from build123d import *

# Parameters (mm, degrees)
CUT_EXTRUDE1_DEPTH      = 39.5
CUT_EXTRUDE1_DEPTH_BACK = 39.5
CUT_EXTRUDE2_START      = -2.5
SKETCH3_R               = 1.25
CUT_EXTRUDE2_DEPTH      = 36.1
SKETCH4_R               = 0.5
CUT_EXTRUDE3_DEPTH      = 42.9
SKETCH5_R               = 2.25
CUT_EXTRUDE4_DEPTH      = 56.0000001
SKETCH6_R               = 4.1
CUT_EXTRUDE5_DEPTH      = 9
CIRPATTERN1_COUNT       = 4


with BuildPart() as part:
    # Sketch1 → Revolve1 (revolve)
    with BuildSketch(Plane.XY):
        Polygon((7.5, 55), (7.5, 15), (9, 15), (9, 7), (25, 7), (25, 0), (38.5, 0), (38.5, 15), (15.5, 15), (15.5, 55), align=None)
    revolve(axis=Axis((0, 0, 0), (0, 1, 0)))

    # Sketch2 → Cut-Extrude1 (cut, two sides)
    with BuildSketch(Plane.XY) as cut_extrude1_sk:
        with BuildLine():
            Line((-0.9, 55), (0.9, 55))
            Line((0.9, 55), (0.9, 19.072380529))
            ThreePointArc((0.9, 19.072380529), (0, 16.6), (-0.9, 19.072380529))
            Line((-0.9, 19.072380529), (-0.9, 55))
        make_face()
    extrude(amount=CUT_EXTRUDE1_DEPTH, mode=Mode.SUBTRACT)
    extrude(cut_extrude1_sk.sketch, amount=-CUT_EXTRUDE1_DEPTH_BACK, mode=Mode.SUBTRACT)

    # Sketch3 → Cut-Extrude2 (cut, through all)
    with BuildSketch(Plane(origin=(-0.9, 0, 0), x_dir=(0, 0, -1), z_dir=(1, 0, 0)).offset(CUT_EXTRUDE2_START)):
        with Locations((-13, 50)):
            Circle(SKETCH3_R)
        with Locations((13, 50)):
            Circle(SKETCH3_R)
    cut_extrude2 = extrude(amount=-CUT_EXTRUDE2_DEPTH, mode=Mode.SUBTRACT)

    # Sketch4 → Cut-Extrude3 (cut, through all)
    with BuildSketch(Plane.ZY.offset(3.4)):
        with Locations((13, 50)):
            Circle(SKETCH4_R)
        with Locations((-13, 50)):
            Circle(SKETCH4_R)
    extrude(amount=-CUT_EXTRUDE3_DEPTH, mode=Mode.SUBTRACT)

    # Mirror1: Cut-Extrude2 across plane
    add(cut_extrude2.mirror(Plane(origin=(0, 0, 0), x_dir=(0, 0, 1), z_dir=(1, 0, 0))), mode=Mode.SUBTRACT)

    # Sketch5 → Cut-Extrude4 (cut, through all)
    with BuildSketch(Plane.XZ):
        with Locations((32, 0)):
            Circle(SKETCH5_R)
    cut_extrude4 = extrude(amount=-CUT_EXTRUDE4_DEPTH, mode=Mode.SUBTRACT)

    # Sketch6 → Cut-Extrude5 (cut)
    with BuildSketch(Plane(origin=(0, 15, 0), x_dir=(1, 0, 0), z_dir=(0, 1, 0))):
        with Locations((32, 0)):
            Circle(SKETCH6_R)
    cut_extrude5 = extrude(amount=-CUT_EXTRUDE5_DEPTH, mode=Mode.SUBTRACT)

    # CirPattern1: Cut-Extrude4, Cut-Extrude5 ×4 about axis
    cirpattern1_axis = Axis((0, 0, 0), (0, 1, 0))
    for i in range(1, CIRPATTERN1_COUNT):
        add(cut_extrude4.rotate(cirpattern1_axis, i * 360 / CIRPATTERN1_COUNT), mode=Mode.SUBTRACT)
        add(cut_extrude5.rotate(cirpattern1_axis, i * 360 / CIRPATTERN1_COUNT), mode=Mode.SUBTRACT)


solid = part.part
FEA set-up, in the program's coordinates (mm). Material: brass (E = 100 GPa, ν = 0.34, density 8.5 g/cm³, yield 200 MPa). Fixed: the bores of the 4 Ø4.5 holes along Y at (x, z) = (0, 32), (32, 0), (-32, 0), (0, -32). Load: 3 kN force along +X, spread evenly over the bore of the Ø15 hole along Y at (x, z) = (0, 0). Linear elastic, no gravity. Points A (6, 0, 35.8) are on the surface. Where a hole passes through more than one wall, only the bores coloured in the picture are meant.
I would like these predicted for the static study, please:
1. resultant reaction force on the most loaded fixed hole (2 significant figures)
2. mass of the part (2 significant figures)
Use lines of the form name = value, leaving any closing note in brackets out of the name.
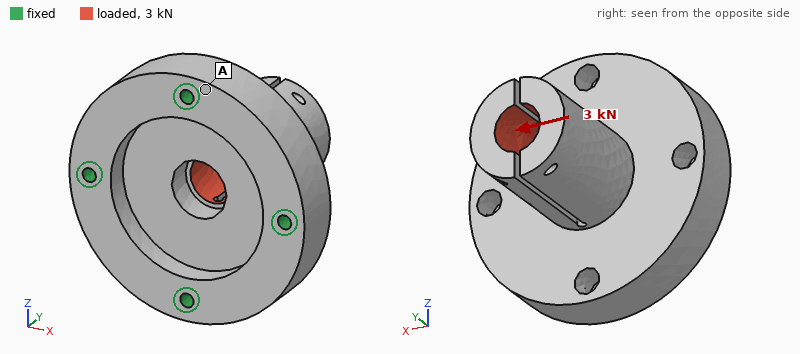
resultant reaction force on the most loaded fixed hole = 1.9 kN
mass of the part = 630 g
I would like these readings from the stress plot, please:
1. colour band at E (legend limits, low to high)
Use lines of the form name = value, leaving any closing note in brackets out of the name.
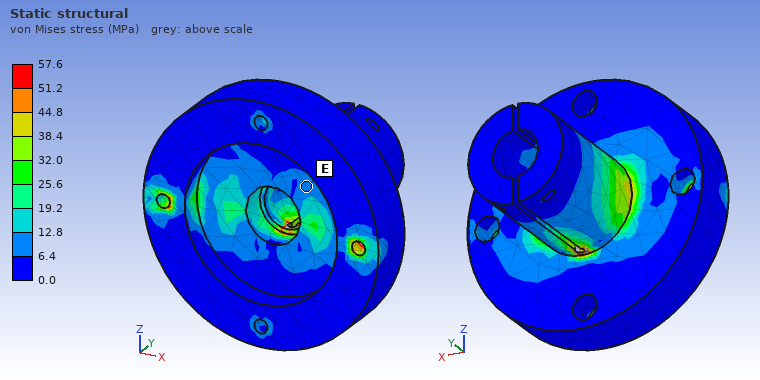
colour band at E = 6.4 to 12.8 MPa
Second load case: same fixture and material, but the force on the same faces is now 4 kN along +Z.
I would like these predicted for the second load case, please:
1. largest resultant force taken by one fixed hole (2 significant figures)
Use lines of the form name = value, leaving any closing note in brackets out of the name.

largest resultant force taken by one fixed hole = 2.6 kN
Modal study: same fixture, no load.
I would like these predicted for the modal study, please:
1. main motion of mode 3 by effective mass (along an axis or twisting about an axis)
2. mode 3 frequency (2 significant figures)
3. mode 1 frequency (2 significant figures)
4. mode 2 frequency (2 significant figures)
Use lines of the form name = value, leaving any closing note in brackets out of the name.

main motion of mode 3 by effective mass = along Z
mode 3 frequency = 4000 Hz
mode 1 frequency = 3100 Hz
mode 2 frequency = 3200 Hz
